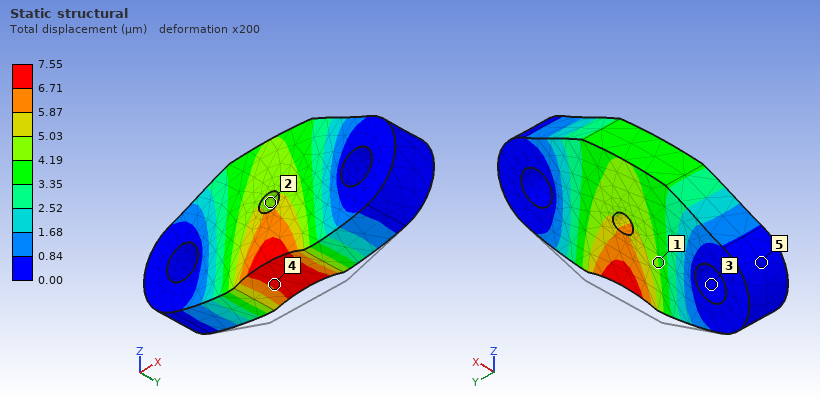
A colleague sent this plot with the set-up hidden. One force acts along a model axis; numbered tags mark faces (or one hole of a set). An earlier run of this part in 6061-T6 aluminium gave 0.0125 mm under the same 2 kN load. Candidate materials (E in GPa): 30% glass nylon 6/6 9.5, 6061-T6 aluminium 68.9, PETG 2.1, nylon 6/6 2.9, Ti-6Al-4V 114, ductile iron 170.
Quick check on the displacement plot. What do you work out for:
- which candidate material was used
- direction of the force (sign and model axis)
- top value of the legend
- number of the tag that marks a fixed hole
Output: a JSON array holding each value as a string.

["Ti-6Al-4V", "+Z", "7.55 µm", "3"]
